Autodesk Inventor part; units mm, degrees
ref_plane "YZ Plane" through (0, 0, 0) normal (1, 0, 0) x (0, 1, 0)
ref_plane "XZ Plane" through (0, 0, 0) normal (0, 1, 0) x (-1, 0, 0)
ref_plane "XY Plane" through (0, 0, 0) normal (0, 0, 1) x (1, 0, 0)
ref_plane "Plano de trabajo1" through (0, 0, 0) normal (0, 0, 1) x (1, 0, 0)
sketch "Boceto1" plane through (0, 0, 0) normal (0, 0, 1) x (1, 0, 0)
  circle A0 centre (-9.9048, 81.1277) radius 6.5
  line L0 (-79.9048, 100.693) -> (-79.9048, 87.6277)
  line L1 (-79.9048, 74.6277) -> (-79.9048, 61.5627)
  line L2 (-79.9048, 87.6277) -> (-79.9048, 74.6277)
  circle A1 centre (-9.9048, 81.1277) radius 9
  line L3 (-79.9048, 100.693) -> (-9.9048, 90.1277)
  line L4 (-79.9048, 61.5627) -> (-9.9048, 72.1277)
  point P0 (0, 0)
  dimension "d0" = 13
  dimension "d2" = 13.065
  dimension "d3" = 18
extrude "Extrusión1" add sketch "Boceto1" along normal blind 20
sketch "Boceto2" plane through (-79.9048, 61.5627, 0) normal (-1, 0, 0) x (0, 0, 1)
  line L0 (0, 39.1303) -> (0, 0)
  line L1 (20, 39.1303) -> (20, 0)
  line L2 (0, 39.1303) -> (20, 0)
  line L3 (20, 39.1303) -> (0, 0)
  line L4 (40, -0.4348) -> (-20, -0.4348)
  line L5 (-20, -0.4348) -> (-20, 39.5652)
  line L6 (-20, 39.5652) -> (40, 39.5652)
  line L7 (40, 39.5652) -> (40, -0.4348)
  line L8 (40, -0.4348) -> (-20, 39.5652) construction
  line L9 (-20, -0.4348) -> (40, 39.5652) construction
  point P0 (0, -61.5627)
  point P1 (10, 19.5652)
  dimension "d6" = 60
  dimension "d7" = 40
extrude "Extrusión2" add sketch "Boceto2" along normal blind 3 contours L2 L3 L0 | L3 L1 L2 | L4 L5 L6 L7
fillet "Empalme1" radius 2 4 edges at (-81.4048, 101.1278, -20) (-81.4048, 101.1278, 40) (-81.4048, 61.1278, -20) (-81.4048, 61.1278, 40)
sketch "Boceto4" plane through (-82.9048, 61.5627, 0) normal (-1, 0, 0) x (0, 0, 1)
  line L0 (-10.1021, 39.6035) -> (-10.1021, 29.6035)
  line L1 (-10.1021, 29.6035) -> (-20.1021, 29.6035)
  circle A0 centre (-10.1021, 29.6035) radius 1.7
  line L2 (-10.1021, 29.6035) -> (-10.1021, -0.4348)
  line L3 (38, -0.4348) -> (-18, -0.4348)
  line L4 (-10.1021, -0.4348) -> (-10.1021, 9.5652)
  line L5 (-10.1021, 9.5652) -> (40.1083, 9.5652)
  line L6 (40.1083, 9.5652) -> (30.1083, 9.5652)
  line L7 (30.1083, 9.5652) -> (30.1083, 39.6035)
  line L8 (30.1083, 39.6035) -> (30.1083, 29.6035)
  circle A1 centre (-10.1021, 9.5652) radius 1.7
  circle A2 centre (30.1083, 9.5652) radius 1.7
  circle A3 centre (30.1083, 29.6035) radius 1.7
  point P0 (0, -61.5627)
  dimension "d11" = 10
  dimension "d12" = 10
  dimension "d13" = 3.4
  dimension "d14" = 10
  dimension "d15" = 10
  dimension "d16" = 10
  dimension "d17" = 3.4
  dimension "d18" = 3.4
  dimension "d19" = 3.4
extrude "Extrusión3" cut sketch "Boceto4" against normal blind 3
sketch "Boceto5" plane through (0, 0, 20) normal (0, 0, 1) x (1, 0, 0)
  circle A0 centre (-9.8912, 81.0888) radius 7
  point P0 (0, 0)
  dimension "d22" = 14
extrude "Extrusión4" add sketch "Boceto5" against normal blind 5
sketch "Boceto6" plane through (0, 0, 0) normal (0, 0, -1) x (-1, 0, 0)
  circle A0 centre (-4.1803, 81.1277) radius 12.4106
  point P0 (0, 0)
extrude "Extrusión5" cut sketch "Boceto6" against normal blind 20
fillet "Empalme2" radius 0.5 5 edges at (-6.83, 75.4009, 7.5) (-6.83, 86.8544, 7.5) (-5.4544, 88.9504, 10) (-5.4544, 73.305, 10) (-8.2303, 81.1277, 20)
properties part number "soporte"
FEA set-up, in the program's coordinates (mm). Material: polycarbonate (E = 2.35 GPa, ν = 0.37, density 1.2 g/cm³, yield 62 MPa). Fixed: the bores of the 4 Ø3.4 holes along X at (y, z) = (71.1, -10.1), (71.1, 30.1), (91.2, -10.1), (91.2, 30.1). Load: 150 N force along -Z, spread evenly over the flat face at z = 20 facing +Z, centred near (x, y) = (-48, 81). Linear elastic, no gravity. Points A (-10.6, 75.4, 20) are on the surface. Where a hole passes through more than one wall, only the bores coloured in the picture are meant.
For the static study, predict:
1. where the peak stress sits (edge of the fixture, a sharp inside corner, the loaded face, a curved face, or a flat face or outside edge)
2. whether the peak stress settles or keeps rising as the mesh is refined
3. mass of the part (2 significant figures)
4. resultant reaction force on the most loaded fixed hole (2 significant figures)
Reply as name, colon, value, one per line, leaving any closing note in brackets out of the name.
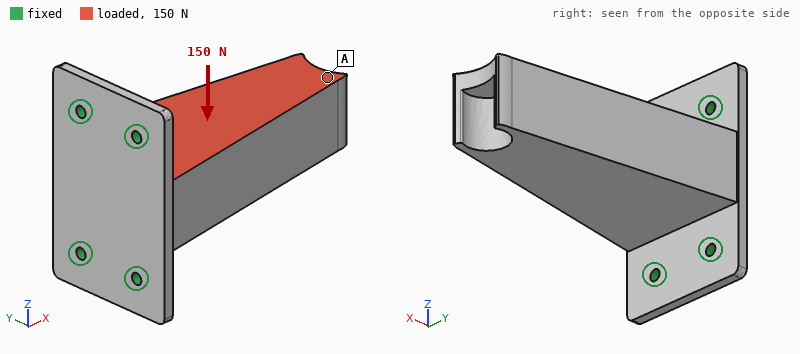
where the peak stress sits: edge of the fixture
whether the peak stress settles or keeps rising as the mesh is refined: keeps rising
mass of the part: 56 g
resultant reaction force on the most loaded fixed hole: 88 N
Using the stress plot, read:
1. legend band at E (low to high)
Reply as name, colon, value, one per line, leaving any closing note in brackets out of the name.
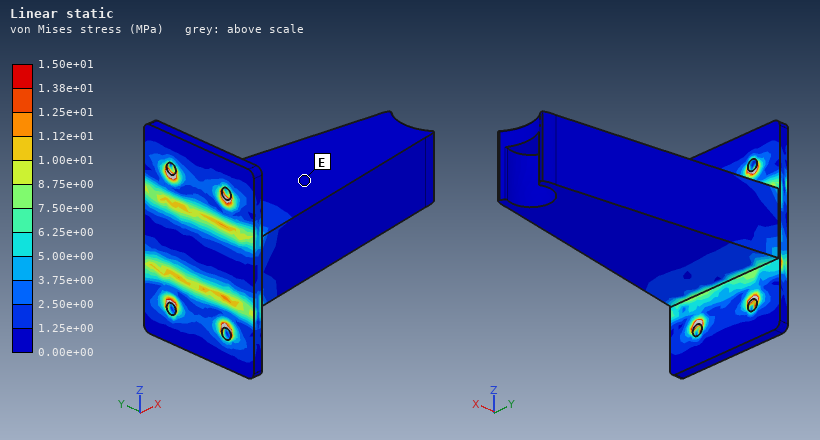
legend band at E: 0.00e+00 to 1.25e+00 MPa
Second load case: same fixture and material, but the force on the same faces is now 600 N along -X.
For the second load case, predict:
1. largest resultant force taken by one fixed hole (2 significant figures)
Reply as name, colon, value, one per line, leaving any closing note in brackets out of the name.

largest resultant force taken by one fixed hole: 260 N
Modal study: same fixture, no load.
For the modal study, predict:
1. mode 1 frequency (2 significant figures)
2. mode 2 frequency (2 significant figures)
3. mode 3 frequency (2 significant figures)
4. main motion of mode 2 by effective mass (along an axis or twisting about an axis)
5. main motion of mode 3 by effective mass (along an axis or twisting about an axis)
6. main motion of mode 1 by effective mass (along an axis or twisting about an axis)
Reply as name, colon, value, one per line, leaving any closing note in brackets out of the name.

mode 1 frequency: 330 Hz
mode 2 frequency: 430 Hz
mode 3 frequency: 1100 Hz
main motion of mode 2 by effective mass: along Z
main motion of mode 3 by effective mass: along X
main motion of mode 1 by effective mass: along Y
